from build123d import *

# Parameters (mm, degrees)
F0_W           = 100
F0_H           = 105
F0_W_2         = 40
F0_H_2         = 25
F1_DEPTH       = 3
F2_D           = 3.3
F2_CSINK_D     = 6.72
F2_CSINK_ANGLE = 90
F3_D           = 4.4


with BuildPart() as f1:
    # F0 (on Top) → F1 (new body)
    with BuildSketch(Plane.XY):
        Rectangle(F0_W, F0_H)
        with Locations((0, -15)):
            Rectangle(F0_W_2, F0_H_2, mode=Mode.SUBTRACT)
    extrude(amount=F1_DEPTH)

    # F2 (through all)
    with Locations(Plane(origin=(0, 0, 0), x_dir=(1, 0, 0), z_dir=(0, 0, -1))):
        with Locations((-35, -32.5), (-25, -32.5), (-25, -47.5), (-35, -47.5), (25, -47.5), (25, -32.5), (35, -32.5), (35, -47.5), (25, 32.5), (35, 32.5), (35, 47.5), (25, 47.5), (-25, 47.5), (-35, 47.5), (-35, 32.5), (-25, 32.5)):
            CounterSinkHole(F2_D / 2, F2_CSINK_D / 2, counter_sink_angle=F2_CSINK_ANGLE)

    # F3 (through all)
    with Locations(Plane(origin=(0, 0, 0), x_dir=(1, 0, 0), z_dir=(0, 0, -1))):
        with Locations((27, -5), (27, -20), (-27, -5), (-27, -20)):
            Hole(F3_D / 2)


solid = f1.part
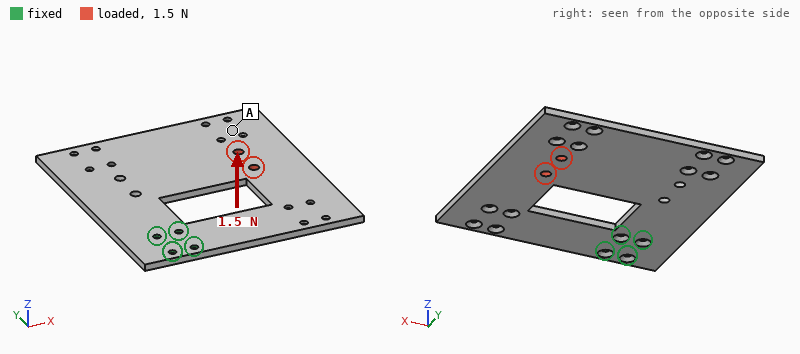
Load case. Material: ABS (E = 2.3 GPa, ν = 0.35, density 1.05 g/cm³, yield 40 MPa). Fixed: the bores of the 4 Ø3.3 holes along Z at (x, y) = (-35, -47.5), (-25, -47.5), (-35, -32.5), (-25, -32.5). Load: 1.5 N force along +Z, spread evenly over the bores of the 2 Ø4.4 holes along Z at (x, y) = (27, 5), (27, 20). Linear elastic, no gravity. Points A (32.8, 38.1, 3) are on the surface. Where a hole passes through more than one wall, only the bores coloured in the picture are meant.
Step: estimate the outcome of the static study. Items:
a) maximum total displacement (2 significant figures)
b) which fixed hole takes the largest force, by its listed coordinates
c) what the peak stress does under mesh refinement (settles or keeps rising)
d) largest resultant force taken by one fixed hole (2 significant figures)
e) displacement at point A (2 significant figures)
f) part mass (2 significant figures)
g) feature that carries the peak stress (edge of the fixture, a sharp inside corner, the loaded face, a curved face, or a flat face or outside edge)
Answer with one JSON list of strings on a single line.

["1.5 mm", "(-25, -32.5)", "keeps rising", "8.6 N", "1.1 mm", "29 g", "edge of the fixture"]
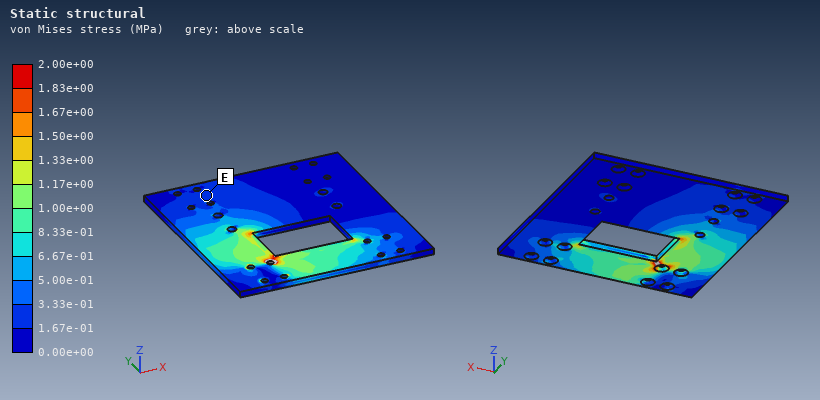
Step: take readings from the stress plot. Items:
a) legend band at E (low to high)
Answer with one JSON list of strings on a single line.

["1.67e-01 to 3.33e-01 MPa"]
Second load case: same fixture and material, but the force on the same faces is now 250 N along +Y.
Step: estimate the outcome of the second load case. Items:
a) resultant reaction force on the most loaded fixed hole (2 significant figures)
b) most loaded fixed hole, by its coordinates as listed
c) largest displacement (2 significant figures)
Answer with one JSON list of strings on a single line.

["550 N", "(-25, -32.5)", "1.7 mm"]
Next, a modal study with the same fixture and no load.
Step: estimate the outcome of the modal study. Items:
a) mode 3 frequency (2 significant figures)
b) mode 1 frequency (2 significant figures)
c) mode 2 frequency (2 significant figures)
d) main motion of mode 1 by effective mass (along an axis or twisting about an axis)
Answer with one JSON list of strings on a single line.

["220 Hz", "53 Hz", "100 Hz", "along Z"]
